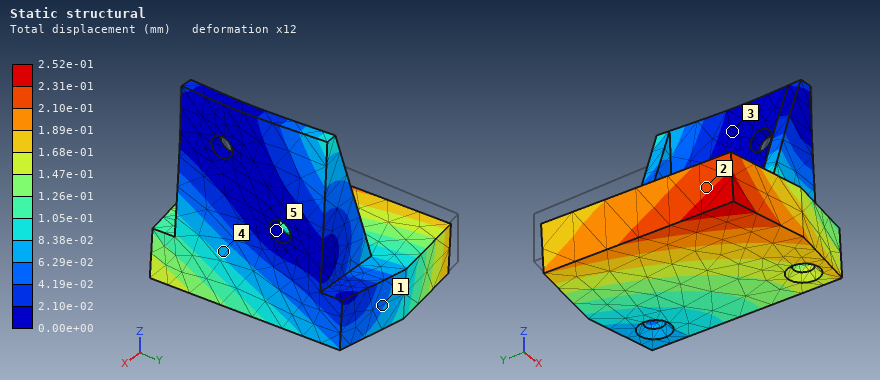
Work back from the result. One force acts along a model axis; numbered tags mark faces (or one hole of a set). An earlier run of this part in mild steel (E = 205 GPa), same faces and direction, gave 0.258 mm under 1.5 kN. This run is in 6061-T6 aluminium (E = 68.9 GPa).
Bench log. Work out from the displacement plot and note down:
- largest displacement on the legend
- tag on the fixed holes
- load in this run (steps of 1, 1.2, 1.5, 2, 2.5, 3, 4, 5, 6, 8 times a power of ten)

2.52e-01 mm
5
500 N
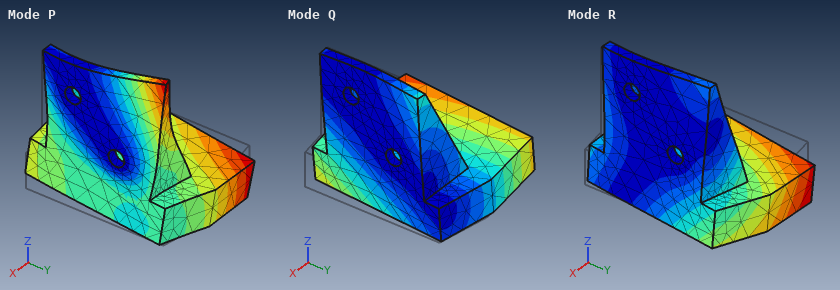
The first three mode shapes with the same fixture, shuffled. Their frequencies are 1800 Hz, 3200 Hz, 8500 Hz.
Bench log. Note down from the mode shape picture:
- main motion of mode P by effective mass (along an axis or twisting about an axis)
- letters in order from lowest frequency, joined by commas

along X
Q, R, P
